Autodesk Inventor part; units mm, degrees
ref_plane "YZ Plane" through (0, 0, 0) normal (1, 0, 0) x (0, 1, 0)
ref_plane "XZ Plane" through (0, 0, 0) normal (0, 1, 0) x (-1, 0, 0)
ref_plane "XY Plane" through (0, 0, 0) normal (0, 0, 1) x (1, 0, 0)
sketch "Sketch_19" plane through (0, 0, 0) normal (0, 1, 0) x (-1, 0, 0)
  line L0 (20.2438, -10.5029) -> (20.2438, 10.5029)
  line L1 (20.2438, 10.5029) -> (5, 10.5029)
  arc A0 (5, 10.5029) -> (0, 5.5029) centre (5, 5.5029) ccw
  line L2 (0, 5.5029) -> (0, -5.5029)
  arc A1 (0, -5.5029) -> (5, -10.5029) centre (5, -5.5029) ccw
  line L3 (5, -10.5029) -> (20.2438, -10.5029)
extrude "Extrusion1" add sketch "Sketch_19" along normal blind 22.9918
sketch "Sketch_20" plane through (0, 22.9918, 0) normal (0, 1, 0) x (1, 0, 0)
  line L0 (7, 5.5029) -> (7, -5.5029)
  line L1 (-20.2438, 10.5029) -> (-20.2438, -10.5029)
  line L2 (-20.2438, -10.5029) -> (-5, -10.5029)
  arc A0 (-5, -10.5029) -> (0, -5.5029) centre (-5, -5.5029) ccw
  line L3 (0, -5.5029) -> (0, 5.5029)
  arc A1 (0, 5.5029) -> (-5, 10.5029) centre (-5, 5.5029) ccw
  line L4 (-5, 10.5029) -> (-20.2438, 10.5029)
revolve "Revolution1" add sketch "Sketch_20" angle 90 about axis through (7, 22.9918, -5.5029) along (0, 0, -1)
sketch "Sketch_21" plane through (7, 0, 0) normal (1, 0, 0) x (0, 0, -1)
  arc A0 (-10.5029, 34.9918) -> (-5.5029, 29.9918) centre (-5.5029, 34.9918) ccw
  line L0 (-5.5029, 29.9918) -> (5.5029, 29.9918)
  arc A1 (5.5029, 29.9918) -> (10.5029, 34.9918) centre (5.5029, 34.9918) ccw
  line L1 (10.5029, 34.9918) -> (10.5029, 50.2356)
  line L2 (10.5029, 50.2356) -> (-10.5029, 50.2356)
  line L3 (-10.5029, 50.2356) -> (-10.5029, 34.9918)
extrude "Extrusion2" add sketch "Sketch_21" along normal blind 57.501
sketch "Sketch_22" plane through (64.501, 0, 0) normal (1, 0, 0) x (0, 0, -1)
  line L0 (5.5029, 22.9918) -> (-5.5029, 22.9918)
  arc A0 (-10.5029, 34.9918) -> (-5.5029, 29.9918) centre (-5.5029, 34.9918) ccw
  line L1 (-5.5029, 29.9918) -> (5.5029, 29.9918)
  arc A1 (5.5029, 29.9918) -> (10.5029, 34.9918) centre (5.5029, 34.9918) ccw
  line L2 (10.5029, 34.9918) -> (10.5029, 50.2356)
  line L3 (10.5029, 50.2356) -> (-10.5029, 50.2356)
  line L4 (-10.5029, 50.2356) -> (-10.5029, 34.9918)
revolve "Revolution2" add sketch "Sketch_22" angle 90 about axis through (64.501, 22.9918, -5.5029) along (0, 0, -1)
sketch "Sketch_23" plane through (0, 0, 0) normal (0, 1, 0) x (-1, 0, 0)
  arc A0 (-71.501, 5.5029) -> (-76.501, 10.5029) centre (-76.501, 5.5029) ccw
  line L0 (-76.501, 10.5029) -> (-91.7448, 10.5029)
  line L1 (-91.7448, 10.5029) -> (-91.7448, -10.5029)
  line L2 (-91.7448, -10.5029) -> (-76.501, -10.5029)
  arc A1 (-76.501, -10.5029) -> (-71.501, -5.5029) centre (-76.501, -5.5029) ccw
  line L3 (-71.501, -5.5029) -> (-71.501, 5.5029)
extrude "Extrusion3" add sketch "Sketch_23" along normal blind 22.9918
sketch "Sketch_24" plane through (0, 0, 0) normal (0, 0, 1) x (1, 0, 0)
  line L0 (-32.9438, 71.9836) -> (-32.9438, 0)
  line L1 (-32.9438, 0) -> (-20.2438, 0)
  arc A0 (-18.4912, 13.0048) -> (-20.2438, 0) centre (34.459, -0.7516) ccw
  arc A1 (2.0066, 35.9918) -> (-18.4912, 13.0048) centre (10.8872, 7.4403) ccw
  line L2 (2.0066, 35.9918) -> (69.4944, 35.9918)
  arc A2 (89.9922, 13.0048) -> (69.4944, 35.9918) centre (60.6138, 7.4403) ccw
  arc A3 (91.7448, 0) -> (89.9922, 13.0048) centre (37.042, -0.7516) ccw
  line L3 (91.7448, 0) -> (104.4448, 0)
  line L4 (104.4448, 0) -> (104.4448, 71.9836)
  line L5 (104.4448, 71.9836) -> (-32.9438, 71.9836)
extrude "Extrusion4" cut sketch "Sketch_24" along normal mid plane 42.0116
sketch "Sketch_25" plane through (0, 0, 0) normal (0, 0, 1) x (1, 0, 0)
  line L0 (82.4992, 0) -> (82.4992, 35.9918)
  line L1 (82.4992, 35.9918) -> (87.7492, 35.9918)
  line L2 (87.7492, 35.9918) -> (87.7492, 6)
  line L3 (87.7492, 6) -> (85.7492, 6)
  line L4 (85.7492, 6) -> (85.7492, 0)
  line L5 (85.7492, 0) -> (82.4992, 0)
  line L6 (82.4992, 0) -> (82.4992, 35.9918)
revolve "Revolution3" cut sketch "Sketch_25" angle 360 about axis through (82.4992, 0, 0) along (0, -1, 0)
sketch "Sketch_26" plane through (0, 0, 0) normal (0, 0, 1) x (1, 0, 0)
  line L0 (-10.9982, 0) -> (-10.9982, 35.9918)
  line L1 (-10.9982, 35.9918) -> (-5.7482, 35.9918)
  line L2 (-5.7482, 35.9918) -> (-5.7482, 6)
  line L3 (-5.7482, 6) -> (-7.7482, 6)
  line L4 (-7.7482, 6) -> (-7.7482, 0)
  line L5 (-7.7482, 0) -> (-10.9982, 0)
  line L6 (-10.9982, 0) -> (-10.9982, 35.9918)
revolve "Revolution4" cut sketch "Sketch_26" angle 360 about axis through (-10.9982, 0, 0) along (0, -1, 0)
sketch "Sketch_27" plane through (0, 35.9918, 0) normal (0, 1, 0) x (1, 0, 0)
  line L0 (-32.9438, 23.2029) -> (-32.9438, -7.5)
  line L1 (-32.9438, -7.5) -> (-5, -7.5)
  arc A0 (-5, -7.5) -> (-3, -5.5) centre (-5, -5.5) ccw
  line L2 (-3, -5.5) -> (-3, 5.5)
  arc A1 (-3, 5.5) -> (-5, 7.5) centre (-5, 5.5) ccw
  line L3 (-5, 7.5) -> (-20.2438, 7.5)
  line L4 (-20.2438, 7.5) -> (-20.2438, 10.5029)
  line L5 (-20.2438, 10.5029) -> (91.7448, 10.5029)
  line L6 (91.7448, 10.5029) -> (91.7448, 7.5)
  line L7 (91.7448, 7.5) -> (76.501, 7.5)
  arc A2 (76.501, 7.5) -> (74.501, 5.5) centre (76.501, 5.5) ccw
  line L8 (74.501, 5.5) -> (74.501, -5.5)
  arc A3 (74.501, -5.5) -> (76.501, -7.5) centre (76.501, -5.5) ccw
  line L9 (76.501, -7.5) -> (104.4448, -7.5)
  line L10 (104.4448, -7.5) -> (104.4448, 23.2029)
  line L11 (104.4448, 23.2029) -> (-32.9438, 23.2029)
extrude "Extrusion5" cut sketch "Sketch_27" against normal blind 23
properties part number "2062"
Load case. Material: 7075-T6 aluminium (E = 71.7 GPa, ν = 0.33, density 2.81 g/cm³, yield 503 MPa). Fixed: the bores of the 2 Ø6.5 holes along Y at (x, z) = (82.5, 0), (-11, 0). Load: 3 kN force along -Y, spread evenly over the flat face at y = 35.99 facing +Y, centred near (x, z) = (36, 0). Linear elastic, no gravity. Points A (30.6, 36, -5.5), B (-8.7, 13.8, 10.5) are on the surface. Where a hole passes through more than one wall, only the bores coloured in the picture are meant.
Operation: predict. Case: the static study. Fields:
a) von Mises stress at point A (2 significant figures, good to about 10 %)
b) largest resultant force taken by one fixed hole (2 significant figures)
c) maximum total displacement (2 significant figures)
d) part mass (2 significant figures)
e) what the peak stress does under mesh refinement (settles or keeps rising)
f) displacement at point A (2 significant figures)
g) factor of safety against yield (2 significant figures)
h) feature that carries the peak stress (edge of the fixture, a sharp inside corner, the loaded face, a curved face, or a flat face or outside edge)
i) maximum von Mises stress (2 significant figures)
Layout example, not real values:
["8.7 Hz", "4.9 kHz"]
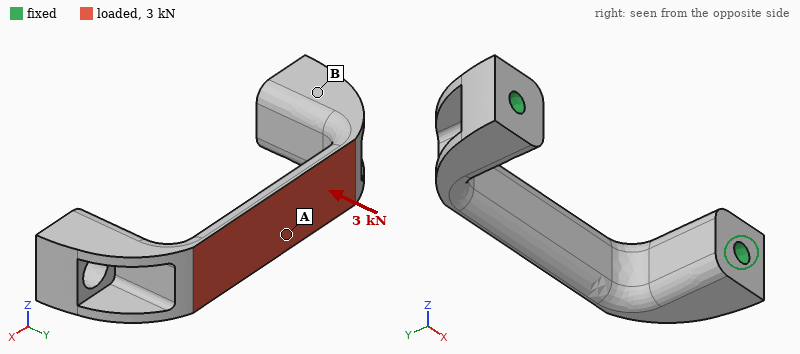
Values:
["100 MPa", "1.9 kN", "0.20 mm", "63 g", "settles", "0.19 mm", "3.1", "a curved face", "160 MPa"]
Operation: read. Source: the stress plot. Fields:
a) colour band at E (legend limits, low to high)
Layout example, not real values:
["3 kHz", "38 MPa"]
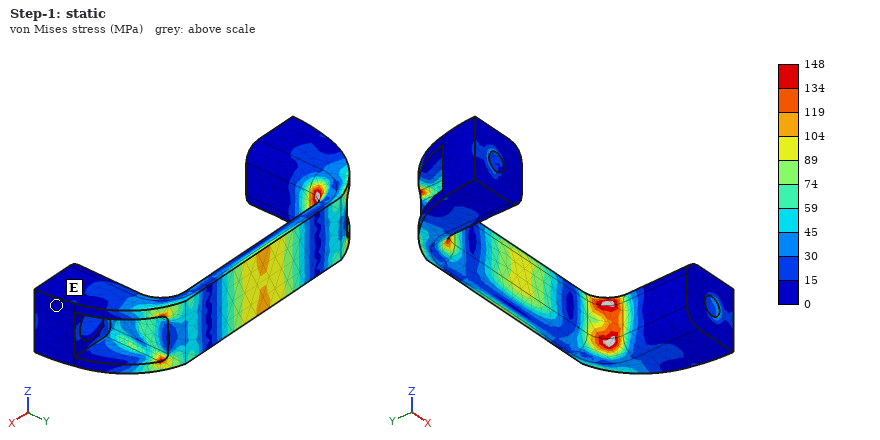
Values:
["0 to 15 MPa"]
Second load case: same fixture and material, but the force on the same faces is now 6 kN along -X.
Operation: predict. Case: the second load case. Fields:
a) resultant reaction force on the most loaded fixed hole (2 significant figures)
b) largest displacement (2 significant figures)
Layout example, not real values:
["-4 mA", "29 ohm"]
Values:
["3.1 kN", "0.21 mm"]
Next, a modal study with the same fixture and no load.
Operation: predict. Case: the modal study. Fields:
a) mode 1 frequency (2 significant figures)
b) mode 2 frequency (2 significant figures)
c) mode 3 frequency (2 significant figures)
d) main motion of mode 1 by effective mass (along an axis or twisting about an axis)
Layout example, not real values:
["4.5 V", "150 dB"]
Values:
["4000 Hz", "4800 Hz", "4800 Hz", "along Z"]
